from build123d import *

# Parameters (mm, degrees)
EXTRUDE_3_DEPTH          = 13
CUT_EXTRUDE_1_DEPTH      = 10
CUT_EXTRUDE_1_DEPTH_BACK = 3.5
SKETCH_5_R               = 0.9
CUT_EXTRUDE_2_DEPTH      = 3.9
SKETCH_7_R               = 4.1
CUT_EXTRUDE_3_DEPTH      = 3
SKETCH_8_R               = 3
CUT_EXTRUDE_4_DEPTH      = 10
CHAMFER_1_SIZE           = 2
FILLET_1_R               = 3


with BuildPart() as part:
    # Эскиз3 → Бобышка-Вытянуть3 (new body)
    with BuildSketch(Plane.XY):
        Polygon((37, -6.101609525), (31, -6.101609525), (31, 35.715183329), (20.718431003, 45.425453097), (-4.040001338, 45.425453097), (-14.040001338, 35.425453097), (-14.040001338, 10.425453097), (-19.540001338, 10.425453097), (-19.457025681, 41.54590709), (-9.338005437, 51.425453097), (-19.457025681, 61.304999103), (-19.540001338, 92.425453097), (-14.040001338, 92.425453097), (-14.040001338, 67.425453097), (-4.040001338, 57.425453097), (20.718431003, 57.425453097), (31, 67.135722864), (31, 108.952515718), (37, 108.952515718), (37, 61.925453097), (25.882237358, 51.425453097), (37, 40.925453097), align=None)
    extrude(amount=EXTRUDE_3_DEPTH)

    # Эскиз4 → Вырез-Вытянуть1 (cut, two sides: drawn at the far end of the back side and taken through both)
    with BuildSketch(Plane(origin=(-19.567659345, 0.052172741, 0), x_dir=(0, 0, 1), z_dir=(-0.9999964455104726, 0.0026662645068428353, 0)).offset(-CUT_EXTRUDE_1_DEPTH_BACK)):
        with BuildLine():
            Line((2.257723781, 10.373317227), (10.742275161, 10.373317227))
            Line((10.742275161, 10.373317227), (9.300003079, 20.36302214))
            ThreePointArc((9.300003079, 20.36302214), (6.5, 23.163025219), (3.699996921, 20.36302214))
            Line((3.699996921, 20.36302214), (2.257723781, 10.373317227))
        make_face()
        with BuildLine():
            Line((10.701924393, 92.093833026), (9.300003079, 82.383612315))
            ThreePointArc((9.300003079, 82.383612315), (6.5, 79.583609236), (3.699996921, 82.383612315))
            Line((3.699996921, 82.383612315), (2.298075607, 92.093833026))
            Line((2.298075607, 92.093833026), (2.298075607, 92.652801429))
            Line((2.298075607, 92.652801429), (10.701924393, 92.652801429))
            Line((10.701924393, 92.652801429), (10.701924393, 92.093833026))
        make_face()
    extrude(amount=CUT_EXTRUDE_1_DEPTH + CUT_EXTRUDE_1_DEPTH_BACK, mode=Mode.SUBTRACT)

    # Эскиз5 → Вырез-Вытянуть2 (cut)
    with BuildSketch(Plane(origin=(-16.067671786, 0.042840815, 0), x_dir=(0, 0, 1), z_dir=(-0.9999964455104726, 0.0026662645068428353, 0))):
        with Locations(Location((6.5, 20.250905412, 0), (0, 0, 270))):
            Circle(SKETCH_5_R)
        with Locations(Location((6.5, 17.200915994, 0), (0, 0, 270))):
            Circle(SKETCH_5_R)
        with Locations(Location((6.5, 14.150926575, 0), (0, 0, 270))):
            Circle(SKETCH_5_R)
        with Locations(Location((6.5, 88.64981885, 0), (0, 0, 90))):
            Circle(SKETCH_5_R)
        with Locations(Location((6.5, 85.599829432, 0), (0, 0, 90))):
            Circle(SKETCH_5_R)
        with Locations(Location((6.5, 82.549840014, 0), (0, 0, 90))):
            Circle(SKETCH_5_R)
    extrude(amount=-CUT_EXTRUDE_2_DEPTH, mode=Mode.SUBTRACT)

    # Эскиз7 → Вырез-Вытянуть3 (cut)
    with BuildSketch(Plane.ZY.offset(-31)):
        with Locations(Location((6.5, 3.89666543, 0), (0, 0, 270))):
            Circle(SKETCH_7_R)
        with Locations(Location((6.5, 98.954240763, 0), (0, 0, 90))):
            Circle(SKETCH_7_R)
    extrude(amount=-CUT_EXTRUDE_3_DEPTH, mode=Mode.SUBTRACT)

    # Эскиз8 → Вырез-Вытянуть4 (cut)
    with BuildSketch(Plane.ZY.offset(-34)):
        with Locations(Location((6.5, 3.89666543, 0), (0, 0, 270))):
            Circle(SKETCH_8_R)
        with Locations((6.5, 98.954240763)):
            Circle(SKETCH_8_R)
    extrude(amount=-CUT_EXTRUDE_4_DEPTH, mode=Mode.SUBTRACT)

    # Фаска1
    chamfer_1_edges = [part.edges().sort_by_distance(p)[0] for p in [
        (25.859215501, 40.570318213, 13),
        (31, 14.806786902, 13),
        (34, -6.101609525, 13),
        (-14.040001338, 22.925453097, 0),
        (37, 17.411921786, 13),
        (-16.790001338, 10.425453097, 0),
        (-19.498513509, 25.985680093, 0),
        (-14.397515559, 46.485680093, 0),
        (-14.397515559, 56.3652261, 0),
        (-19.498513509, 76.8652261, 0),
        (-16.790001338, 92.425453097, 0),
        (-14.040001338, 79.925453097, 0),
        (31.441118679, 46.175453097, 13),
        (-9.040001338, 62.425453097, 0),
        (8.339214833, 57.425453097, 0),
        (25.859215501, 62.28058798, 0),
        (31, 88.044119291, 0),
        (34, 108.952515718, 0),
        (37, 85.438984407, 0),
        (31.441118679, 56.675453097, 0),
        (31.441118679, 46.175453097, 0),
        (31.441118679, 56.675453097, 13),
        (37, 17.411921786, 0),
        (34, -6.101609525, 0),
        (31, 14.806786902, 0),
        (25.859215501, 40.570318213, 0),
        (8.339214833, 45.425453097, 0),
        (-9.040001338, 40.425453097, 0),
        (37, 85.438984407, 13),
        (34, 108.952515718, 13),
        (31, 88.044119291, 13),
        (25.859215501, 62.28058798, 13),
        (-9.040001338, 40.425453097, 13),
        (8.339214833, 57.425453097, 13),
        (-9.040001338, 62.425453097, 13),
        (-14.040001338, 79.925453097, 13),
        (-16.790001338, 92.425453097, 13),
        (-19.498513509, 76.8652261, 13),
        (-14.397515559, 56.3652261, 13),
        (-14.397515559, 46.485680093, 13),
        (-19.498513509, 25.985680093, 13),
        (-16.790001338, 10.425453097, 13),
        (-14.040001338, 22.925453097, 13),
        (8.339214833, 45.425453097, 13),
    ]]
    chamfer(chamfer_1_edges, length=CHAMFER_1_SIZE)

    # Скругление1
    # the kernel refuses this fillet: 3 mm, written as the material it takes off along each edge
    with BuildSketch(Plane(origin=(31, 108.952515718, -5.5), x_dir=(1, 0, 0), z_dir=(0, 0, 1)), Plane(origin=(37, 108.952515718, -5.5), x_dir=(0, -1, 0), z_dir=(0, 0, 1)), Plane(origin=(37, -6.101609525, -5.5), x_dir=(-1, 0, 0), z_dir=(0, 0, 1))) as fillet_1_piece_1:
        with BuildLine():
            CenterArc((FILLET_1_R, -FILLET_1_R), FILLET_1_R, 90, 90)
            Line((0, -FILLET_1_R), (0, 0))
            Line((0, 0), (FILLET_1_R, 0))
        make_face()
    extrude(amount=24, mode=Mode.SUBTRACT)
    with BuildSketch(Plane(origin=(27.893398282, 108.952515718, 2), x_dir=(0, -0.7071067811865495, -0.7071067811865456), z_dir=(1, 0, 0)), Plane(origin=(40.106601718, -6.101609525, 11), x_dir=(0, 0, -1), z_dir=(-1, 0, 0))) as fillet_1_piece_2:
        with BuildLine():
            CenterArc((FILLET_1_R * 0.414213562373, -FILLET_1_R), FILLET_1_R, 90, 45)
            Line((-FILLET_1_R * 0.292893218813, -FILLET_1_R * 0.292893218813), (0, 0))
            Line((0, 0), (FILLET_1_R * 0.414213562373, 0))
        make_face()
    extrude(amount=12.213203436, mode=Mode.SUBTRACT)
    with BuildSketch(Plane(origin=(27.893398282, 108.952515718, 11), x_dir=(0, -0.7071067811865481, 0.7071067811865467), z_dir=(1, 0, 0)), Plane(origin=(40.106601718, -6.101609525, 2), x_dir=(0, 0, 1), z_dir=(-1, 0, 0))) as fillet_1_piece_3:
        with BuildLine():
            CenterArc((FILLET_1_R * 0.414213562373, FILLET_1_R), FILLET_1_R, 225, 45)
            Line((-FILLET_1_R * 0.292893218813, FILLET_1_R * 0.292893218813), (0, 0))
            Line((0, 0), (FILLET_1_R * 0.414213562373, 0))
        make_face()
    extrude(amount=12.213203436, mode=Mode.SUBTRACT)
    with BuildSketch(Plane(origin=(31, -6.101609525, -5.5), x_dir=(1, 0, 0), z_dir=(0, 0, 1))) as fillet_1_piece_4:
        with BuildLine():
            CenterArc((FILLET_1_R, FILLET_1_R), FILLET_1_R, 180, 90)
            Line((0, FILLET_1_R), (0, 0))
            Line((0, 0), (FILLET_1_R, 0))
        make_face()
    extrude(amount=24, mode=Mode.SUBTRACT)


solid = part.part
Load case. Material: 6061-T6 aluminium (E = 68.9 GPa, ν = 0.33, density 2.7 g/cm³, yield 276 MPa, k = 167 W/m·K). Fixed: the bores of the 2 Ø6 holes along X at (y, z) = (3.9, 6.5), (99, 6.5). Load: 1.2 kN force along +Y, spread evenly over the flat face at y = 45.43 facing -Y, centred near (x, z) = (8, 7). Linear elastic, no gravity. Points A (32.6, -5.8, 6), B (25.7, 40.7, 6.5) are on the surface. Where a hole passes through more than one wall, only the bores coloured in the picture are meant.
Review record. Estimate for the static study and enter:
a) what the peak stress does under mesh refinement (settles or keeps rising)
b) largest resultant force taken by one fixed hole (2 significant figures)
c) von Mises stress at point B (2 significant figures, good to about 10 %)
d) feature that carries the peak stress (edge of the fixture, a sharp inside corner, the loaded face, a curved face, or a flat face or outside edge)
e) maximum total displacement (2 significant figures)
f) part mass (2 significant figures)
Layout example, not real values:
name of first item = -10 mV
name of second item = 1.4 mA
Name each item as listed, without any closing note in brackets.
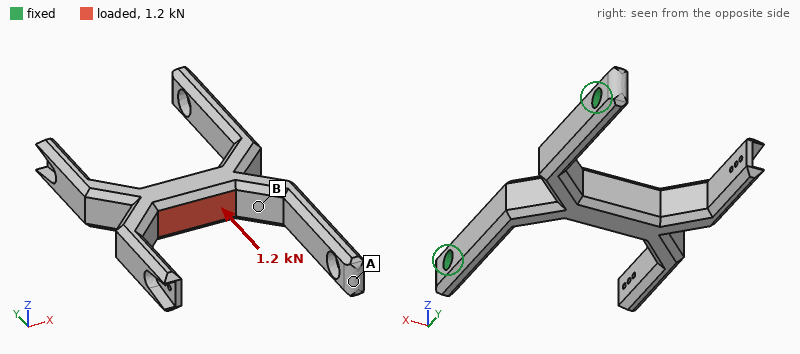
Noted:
what the peak stress does under mesh refinement = keeps rising
largest resultant force taken by one fixed hole = 750 N
von Mises stress at point B = 83 MPa
feature that carries the peak stress = edge of the fixture
maximum total displacement = 0.54 mm
part mass = 50 g
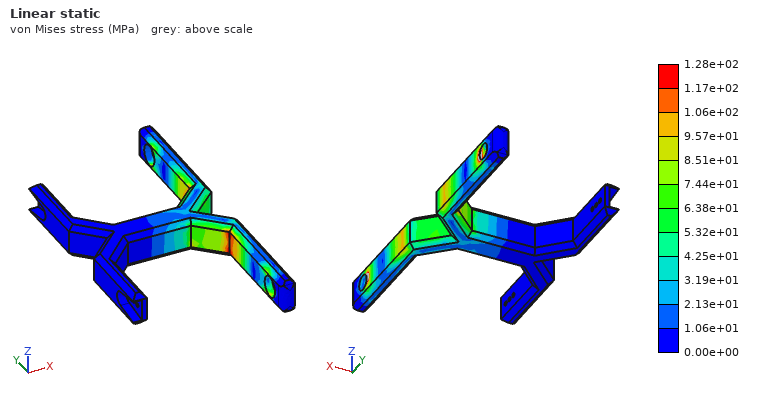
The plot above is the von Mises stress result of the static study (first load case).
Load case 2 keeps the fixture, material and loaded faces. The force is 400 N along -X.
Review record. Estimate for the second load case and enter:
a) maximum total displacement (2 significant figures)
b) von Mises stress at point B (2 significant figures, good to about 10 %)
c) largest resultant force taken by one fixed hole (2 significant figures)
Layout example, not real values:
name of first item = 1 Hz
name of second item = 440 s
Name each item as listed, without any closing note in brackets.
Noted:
maximum total displacement = 0.12 mm
von Mises stress at point B = 28 MPa
largest resultant force taken by one fixed hole = 550 N
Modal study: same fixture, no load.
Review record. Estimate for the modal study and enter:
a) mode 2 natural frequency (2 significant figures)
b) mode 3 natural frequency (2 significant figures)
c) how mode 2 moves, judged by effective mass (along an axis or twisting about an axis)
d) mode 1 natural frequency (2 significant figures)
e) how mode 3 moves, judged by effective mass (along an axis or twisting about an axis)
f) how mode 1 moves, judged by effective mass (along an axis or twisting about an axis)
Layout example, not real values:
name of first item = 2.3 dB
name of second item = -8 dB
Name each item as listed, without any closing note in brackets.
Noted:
mode 2 natural frequency = 1300 Hz
mode 3 natural frequency = 1900 Hz
how mode 2 moves, judged by effective mass = along Y
mode 1 natural frequency = 630 Hz
how mode 3 moves, judged by effective mass = along X
how mode 1 moves, judged by effective mass = along Z
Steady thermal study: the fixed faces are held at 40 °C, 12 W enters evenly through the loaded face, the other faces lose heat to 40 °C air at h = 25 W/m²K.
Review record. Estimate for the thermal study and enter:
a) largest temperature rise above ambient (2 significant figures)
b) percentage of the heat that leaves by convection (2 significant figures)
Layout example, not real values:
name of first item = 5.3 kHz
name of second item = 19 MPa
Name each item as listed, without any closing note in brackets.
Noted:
largest temperature rise above ambient = 24 K
percentage of the heat that leaves by convection = 25 %
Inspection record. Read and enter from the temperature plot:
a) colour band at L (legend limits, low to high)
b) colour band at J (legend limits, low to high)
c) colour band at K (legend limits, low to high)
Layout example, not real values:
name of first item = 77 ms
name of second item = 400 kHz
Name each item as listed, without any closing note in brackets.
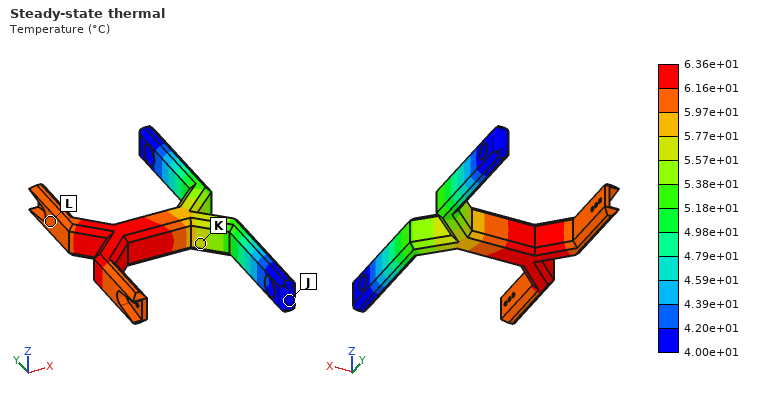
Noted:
colour band at L = 5.97e+01 to 6.16e+01 °C
colour band at J = 4.00e+01 to 4.20e+01 °C
colour band at K = 5.57e+01 to 5.77e+01 °C
